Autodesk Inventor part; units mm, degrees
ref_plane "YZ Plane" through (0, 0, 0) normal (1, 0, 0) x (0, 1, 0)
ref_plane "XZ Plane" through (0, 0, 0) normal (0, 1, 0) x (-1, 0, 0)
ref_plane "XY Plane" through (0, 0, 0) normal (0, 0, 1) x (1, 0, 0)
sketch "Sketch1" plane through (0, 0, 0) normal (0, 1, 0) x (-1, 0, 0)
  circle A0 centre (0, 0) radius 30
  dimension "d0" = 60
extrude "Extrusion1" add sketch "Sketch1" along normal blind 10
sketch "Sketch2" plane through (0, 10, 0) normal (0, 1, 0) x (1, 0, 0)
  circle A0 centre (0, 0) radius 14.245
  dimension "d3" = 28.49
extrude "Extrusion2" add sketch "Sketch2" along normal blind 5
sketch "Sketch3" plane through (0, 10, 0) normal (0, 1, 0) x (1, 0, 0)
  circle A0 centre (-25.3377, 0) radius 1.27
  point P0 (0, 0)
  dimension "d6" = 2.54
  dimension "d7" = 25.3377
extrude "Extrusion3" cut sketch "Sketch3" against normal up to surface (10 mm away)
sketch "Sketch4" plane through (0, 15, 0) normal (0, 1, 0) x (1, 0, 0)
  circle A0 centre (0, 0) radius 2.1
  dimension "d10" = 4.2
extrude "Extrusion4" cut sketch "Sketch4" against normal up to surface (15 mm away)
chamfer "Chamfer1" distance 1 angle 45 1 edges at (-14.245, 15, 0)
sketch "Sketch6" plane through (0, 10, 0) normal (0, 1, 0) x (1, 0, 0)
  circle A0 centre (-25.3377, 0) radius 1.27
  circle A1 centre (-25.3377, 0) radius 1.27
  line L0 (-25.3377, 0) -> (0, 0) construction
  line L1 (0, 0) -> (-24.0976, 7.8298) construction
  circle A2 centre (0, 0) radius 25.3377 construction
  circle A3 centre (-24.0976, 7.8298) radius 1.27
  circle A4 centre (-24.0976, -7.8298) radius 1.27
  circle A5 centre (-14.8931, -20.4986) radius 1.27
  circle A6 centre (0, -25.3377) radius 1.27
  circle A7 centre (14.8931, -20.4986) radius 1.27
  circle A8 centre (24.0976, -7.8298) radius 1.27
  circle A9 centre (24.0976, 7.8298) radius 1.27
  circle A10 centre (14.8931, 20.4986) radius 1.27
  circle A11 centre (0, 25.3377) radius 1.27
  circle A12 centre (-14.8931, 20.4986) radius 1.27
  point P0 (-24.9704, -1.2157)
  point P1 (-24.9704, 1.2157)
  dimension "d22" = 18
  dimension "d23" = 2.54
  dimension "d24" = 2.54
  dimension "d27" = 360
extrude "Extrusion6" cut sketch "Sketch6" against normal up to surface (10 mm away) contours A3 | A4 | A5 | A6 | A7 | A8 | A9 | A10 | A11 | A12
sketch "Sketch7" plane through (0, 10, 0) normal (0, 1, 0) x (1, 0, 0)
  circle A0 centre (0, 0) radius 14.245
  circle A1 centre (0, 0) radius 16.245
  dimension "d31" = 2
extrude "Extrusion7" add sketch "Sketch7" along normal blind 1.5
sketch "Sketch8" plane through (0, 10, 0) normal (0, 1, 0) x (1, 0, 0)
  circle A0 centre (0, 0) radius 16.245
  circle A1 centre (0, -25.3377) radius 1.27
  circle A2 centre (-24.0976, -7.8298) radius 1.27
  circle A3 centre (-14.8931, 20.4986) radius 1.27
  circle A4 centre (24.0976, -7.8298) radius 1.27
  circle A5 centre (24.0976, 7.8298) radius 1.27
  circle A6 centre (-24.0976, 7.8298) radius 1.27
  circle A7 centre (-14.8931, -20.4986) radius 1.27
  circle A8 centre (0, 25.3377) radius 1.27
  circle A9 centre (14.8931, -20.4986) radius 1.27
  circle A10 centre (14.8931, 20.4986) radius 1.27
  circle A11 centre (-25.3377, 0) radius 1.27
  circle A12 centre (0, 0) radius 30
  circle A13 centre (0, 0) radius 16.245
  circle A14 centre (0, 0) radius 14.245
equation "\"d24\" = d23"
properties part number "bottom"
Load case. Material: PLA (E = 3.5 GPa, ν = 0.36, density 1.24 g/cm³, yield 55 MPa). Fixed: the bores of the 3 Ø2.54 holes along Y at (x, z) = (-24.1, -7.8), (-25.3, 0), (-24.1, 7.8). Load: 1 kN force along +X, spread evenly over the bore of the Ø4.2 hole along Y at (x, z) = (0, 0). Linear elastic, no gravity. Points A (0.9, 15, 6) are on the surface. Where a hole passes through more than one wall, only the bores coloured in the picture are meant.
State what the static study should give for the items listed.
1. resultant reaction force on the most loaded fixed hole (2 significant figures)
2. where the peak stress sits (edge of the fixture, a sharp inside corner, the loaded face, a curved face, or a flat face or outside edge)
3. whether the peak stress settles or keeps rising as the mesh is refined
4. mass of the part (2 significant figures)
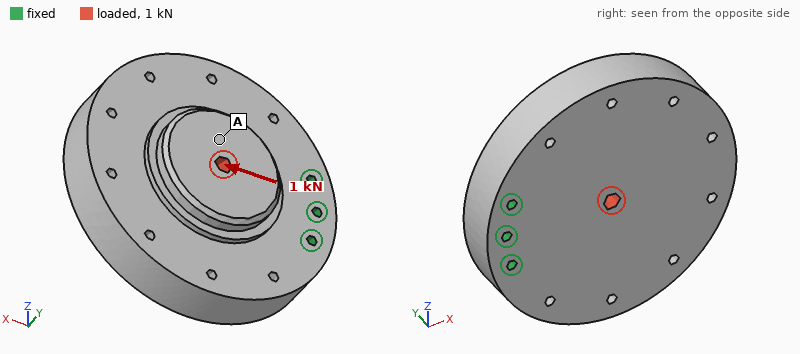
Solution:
380 N
edge of the fixture
keeps rising
38 g
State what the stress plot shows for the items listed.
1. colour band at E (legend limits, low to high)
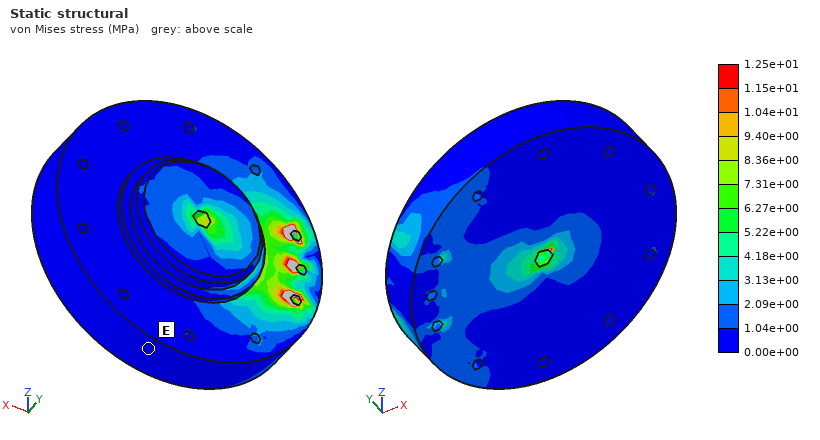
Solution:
0.00e+00 to 1.04e+00 MPa
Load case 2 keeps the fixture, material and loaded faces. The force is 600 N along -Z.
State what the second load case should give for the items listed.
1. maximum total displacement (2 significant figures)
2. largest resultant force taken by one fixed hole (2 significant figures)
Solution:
0.20 mm
860 N
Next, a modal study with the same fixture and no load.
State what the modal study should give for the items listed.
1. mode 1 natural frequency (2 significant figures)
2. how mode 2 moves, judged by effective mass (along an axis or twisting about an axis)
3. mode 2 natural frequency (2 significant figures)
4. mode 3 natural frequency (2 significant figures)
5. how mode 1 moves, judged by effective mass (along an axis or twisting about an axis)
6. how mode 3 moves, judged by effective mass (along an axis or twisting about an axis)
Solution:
860 Hz
along Z
1600 Hz
2000 Hz
along Y
twisting about X
